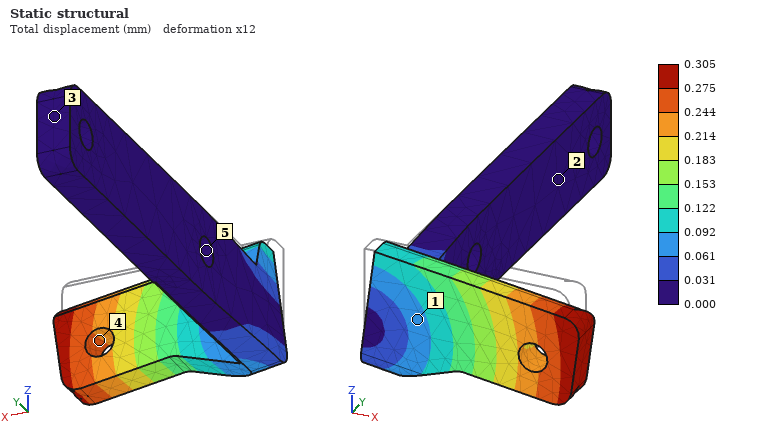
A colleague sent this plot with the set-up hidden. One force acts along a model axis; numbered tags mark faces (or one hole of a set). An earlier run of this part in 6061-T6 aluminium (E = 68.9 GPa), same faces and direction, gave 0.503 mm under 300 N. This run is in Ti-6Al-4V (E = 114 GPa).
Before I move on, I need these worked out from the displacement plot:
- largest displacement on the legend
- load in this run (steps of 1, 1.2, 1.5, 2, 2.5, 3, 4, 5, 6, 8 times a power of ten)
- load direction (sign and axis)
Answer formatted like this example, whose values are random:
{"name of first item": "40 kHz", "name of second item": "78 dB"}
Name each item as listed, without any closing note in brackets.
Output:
{"largest displacement on the legend": "0.305 mm", "load in this run": "300 N", "load direction": "-Z"}
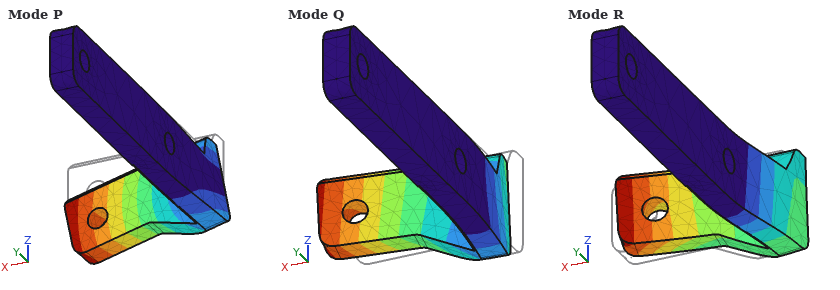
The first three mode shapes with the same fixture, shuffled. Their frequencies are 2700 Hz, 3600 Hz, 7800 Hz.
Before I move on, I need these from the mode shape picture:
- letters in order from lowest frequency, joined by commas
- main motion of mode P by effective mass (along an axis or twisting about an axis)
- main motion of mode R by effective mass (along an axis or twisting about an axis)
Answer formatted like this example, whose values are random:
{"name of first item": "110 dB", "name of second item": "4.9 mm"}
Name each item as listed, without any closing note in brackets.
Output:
{"letters in order from lowest frequency, joined by commas": "Q, P, R", "main motion of mode P by effective mass": "along Z", "main motion of mode R by effective mass": "along X"}
